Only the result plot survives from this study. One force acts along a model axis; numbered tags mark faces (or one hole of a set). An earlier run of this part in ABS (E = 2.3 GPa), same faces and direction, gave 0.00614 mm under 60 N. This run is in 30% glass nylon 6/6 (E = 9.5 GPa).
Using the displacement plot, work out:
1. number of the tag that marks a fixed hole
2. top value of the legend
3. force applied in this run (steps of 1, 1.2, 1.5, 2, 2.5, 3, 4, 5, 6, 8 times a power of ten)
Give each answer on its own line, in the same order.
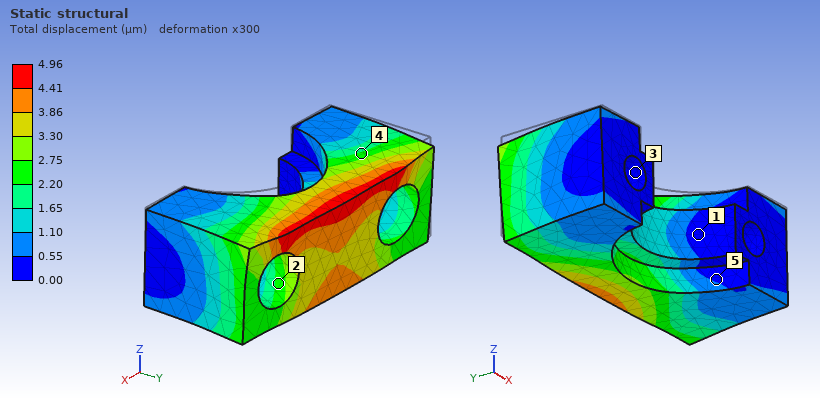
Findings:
3
4.96 µm
200 N
